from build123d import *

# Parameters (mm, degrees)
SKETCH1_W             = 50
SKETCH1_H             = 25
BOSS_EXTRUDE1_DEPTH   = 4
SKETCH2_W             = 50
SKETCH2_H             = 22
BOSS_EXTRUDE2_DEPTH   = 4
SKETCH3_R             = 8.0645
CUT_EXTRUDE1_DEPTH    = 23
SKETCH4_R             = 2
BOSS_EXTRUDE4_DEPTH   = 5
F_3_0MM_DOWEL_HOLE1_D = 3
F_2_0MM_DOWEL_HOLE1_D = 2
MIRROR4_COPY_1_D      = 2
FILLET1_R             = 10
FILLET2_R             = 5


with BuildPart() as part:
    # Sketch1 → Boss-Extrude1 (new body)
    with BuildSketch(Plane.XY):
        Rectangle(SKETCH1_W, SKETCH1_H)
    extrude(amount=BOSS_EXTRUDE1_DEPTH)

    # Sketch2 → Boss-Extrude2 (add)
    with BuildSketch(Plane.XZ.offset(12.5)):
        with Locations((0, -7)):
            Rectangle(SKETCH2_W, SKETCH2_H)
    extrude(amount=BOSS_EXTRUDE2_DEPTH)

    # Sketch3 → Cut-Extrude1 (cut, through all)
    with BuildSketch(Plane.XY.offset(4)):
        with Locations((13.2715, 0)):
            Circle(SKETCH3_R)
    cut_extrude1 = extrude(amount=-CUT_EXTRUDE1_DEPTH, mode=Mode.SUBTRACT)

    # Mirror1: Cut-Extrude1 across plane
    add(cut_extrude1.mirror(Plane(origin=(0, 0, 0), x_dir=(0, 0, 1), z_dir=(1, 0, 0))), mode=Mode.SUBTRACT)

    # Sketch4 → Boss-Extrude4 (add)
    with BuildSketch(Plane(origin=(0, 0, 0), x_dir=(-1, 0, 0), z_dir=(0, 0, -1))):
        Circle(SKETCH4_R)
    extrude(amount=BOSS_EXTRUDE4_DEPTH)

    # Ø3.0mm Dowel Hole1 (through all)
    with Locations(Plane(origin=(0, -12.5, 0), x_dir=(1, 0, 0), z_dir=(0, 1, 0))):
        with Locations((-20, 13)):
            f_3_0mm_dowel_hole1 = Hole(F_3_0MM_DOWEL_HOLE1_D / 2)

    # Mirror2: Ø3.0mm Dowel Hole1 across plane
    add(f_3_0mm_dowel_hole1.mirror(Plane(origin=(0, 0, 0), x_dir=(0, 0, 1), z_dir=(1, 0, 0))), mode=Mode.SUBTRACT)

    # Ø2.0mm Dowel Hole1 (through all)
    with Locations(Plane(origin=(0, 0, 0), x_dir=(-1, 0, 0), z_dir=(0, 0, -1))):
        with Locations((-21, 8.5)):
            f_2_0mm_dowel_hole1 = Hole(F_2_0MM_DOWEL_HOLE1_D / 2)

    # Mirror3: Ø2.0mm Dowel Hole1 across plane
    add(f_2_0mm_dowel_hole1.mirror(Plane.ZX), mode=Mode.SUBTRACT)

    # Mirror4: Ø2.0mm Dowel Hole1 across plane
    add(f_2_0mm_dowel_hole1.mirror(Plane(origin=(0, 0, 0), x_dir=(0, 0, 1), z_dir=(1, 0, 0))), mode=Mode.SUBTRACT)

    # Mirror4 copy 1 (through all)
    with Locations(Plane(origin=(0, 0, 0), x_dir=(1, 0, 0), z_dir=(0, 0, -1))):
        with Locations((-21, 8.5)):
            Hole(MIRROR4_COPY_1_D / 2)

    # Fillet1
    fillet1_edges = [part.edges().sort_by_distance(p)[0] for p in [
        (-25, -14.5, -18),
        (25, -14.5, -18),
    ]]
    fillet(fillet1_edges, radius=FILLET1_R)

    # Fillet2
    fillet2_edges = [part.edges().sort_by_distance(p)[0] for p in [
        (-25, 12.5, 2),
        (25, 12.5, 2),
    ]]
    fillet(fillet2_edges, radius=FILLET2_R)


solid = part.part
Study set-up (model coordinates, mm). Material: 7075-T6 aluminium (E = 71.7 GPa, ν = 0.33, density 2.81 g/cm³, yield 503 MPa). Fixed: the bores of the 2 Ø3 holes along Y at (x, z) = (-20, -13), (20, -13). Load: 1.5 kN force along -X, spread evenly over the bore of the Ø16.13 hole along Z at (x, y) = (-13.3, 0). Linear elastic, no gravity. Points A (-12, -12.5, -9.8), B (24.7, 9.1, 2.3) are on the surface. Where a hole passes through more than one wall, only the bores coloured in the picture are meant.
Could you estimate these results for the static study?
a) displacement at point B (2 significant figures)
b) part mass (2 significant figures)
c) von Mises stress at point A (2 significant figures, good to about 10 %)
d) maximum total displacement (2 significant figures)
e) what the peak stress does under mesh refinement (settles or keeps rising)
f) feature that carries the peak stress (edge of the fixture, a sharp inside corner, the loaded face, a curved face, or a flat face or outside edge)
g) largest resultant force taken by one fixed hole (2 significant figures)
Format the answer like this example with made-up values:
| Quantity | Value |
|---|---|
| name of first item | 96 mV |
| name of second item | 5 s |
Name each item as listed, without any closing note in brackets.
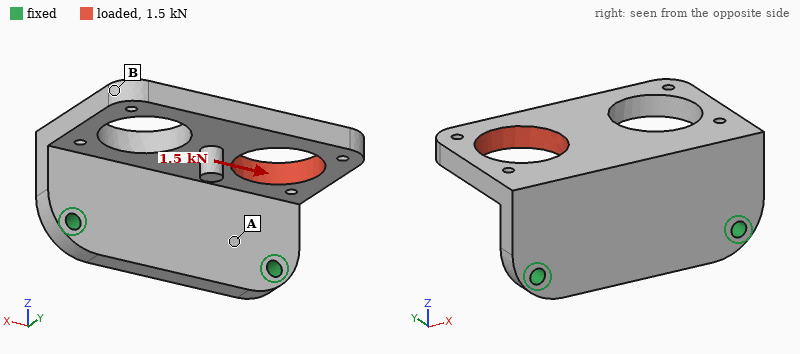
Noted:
| Quantity | Value |
|---|---|
| displacement at point B | 0.14 mm |
| part mass | 21 g |
| von Mises stress at point A | 49 MPa |
| maximum total displacement | 0.15 mm |
| what the peak stress does under mesh refinement | keeps rising |
| feature that carries the peak stress | edge of the fixture |
| largest resultant force taken by one fixed hole | 1.1 kN |
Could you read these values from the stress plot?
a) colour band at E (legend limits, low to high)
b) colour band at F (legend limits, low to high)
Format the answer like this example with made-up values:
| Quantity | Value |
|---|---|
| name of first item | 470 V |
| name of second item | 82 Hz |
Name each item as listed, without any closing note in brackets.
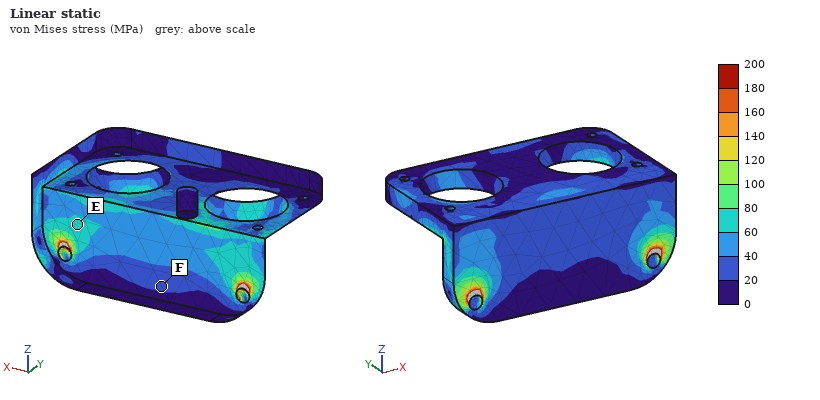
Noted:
| Quantity | Value |
|---|---|
| colour band at E | 60 to 80 MPa |
| colour band at F | 20 to 40 MPa |
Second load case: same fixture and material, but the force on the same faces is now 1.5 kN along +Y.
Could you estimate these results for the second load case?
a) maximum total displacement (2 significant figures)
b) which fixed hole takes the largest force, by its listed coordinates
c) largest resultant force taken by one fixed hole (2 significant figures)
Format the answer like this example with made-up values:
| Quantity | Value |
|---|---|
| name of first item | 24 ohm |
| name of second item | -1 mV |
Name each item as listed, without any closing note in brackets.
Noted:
| Quantity | Value |
|---|---|
| maximum total displacement | 0.50 mm |
| which fixed hole takes the largest force, by its listed coordinates | (-20, -13) |
| largest resultant force taken by one fixed hole | 1.2 kN |
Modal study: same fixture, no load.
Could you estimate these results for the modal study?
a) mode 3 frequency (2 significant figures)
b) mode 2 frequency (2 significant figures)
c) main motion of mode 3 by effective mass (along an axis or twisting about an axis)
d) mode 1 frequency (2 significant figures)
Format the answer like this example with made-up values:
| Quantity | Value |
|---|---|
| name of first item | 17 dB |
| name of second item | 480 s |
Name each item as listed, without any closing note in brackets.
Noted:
| Quantity | Value |
|---|---|
| mode 3 frequency | 6100 Hz |
| mode 2 frequency | 4700 Hz |
| main motion of mode 3 by effective mass | along Y |
| mode 1 frequency | 2300 Hz |
